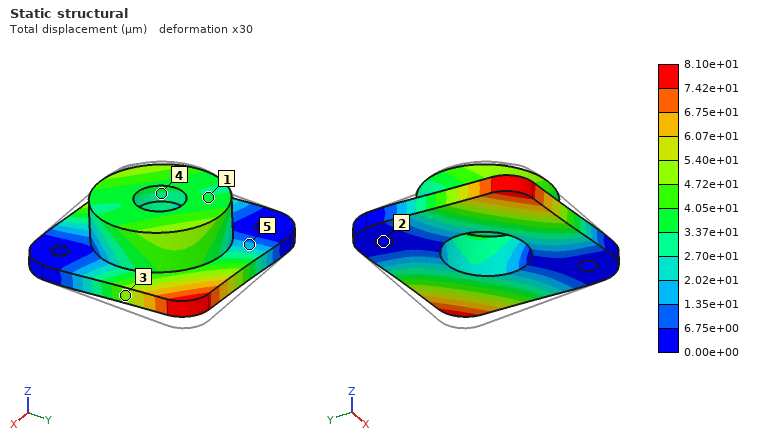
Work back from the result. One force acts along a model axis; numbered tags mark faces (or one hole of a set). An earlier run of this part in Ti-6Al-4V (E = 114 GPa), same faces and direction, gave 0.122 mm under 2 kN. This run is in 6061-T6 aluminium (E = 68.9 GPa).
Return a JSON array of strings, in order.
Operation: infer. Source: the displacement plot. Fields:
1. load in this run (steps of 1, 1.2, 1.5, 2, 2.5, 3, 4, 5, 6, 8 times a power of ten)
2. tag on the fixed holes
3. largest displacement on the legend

["800 N", "2", "8.10e+01 µm"]
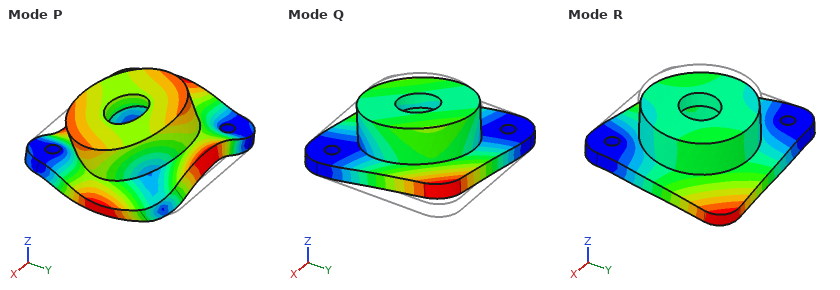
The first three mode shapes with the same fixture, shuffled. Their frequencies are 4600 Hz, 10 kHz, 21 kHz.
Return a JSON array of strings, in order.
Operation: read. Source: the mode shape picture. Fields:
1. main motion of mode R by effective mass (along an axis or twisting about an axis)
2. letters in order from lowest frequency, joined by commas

["along Z", "Q, R, P"]
